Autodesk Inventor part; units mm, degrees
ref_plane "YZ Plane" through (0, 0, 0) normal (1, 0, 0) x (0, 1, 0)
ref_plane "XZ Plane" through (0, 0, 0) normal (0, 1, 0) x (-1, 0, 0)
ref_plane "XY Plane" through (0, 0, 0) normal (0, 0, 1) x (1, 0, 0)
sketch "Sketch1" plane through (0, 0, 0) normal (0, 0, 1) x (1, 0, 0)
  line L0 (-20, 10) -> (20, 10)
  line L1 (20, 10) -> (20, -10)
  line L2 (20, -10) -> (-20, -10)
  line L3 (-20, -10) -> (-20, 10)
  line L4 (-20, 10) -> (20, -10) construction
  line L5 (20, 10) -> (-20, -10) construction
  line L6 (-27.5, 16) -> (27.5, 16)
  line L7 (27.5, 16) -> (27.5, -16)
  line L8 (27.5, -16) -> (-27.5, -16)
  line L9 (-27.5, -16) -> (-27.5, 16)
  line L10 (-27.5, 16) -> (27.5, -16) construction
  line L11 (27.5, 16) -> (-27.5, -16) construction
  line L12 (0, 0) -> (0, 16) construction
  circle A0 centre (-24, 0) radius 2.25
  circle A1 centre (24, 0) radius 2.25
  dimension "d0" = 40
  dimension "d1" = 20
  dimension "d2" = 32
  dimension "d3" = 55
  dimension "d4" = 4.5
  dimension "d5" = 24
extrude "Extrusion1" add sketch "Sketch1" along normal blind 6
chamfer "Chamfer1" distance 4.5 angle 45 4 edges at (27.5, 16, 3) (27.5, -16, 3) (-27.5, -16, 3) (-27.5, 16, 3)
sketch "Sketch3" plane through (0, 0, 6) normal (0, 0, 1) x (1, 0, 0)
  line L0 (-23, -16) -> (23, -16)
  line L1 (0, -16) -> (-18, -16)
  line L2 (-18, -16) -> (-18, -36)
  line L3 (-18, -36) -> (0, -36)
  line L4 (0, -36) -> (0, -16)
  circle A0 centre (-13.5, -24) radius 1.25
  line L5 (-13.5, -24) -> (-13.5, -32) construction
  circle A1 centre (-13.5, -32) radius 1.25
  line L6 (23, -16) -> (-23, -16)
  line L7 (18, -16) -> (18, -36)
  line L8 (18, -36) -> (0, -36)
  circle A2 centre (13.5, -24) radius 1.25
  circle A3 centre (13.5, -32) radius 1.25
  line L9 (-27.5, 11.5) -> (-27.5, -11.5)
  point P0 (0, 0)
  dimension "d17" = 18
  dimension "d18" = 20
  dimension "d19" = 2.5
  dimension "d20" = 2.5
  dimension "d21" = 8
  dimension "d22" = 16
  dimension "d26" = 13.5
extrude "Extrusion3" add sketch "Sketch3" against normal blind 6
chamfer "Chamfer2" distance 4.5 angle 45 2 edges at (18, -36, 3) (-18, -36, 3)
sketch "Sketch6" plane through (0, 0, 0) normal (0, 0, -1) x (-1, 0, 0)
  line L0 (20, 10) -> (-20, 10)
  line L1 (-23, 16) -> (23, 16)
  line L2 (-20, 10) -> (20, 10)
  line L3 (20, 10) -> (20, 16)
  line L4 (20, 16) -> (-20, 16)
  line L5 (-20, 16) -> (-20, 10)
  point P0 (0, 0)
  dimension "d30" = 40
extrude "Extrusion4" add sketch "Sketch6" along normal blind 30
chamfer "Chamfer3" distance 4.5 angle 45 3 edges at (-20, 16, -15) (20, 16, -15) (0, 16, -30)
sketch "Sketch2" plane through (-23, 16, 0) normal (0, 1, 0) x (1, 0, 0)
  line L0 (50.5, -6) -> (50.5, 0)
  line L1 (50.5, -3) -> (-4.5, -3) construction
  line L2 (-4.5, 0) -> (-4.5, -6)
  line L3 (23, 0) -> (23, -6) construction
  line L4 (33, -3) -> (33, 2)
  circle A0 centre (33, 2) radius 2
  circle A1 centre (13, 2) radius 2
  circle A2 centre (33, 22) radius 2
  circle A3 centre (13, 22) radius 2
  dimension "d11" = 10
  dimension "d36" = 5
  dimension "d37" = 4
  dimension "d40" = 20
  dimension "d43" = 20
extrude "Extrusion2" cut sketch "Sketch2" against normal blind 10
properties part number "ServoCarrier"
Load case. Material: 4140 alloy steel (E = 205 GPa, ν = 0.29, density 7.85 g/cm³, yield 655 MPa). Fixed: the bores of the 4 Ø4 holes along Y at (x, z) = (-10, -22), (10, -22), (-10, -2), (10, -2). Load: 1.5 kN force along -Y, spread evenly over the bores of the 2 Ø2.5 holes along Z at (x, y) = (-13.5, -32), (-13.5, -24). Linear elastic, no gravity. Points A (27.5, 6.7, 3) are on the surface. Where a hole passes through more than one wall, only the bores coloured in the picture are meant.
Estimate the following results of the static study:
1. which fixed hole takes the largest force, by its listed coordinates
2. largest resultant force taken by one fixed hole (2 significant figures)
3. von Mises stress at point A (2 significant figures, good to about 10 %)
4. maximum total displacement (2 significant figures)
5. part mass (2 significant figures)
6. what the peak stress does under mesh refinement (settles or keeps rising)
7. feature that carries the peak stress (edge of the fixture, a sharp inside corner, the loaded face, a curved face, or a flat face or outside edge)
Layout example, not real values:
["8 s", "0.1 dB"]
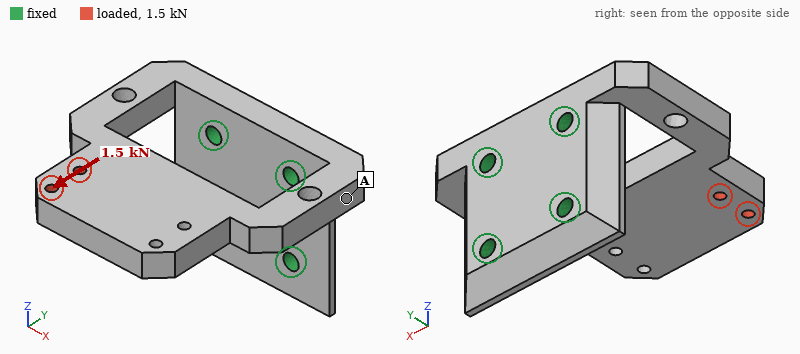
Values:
["(-10, -2)", "1.4 kN", "23 MPa", "51 µm", "120 g", "keeps rising", "edge of the fixture"]
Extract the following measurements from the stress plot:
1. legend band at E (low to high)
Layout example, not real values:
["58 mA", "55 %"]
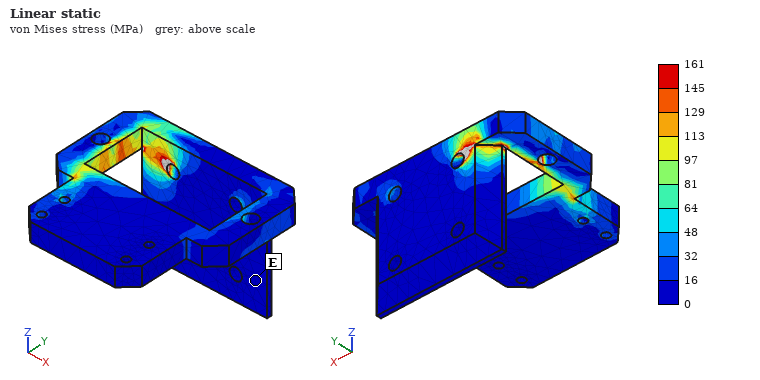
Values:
["0 to 16 MPa"]
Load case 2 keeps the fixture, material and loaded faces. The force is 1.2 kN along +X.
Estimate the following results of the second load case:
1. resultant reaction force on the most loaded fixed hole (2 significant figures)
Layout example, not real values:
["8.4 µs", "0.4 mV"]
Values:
["1.4 kN"]
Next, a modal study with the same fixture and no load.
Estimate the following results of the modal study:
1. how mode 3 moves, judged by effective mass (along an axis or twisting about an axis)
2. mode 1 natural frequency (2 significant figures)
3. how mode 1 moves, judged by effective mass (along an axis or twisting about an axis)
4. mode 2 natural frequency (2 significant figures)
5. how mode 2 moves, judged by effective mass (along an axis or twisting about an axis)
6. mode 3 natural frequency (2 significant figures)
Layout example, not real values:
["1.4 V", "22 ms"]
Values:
["twisting about Y", "900 Hz", "along Z", "2000 Hz", "along X", "3700 Hz"]
